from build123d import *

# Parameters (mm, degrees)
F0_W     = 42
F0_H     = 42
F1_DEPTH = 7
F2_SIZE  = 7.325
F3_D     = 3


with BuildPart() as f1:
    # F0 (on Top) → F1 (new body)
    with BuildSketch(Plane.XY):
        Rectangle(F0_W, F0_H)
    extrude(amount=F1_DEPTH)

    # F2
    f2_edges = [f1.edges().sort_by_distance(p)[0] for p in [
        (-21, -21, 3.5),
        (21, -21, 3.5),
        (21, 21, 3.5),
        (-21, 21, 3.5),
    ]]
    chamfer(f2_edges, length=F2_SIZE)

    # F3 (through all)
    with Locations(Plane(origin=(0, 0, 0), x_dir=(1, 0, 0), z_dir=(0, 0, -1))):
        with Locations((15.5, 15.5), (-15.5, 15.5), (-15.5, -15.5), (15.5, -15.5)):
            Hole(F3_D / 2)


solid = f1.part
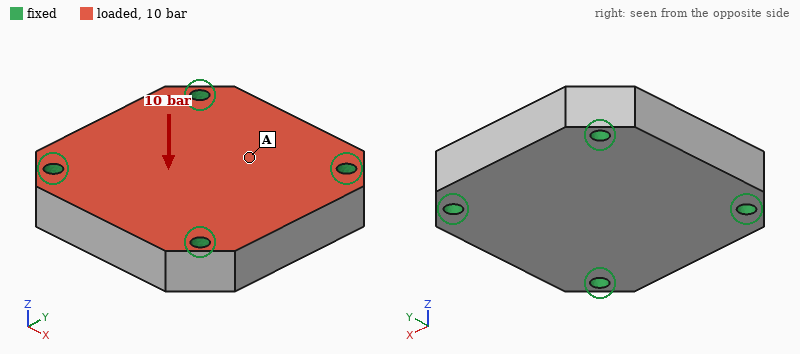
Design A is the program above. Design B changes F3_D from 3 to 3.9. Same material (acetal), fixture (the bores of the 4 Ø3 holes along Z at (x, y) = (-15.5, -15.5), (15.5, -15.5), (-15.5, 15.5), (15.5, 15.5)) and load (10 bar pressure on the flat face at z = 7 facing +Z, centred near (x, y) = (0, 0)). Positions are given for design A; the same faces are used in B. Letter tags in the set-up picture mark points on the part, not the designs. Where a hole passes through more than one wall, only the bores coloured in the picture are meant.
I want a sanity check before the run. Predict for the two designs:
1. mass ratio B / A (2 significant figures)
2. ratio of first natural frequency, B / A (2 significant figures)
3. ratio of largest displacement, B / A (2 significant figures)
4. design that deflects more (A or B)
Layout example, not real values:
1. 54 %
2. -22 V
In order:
1. 0.99
2. 1.1
3. 0.87
4. A
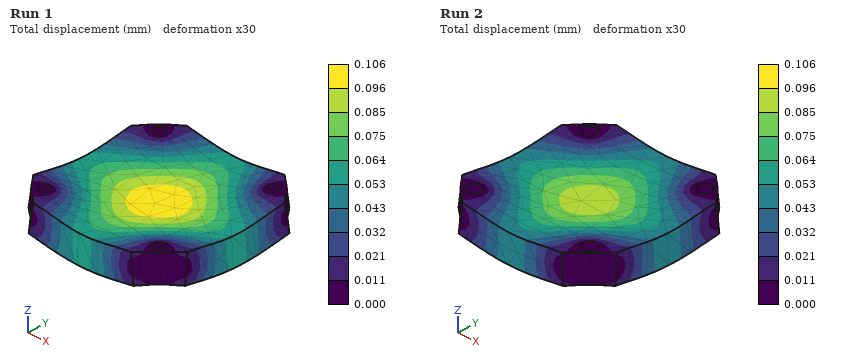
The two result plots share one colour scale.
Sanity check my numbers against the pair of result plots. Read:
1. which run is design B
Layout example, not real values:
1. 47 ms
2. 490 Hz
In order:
1. Run 2
